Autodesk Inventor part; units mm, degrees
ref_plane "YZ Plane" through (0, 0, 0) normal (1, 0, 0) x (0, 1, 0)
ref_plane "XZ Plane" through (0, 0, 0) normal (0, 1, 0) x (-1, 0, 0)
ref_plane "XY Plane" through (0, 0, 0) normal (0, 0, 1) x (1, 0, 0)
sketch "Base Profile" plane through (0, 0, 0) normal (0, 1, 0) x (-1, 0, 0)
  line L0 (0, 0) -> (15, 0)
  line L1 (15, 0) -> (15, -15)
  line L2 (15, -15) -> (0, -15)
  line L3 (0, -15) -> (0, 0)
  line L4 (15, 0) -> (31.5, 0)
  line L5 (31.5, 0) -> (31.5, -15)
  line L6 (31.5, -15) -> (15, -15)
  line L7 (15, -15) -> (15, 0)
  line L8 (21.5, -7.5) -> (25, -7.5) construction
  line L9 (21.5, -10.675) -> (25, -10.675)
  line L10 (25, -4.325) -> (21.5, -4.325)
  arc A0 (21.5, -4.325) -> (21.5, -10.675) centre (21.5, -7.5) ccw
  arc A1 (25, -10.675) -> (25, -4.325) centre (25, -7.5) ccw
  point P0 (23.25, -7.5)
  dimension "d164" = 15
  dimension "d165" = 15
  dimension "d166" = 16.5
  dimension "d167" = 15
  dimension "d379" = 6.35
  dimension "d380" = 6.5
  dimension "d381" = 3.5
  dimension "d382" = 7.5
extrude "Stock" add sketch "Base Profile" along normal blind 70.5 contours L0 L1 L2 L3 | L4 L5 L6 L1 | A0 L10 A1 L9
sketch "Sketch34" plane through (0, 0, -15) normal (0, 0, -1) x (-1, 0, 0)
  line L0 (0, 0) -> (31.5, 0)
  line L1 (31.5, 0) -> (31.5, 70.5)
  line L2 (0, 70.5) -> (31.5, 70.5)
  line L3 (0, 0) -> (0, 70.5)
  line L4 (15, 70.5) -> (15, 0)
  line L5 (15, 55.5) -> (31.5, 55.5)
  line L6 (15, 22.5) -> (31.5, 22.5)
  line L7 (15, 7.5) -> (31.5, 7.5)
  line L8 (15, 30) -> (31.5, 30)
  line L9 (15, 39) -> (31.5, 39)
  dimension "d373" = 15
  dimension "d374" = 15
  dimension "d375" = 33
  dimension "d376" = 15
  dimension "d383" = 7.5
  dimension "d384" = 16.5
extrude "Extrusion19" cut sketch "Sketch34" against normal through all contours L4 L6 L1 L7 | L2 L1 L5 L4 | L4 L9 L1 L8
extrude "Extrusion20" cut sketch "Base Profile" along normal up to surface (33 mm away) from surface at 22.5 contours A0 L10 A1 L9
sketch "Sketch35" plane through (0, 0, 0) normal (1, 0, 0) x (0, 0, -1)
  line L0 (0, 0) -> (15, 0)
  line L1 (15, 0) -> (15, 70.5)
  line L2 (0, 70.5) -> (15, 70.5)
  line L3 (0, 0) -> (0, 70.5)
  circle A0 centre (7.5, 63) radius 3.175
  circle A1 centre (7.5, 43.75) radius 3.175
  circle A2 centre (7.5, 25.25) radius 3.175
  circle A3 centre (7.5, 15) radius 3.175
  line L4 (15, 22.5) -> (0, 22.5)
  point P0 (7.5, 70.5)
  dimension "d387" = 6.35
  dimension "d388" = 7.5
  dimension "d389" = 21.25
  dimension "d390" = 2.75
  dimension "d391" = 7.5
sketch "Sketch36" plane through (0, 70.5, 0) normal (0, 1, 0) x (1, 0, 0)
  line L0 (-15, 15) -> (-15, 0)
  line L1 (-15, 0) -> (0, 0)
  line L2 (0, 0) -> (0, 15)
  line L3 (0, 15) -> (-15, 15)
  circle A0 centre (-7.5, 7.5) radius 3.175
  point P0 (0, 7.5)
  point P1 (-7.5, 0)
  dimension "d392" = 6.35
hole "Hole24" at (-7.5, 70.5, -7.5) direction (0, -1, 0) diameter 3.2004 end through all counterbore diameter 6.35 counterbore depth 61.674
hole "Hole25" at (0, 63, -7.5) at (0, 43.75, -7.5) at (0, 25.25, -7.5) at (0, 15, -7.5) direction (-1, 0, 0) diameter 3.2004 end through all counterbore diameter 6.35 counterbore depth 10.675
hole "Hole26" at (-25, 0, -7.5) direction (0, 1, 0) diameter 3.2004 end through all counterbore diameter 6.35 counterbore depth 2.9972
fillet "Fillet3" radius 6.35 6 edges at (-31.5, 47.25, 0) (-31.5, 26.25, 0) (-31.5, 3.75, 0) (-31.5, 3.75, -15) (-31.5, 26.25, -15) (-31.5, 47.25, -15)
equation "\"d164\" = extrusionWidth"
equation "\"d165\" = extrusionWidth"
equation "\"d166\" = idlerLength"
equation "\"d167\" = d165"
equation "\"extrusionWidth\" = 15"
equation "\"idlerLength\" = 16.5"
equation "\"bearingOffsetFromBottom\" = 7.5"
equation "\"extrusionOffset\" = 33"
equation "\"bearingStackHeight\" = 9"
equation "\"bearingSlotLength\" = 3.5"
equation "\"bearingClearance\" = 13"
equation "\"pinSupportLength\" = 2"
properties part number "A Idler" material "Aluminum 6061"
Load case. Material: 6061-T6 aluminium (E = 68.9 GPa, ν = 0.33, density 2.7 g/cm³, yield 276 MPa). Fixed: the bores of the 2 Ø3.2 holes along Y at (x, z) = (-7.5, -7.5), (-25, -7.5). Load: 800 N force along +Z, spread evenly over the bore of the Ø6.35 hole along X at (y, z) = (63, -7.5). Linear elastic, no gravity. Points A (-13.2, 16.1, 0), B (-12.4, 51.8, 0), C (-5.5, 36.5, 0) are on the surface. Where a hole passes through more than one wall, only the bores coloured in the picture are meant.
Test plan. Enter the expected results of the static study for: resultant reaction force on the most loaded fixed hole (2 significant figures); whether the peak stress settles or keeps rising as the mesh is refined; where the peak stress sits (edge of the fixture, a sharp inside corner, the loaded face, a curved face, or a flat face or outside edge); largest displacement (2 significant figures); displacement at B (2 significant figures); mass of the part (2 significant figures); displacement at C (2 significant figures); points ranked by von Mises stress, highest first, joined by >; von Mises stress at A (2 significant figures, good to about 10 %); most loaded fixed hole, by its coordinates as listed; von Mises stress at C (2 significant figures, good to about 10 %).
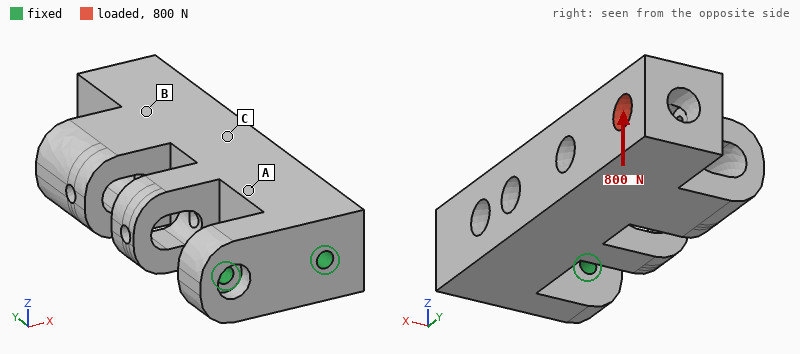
980 N
keeps rising
edge of the fixture
0.41 mm
0.26 mm
51 g
0.16 mm
A > C > B
72 MPa
(-7.5, -7.5)
42 MPa
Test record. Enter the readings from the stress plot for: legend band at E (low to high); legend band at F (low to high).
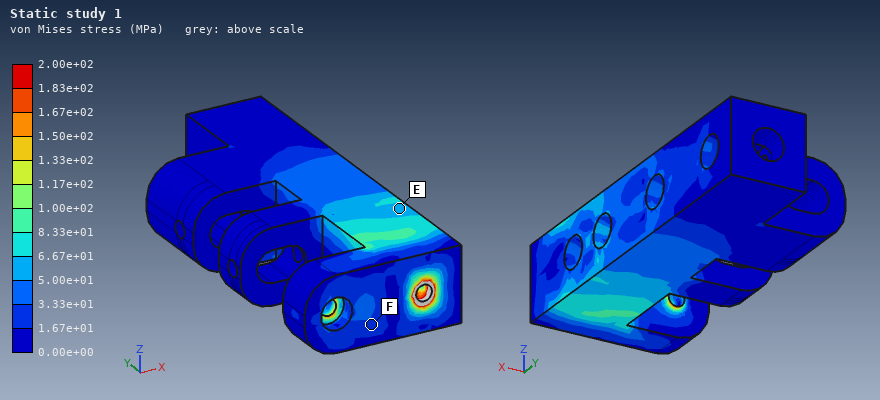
5.00e+01 to 6.67e+01 MPa
1.67e+01 to 3.33e+01 MPa
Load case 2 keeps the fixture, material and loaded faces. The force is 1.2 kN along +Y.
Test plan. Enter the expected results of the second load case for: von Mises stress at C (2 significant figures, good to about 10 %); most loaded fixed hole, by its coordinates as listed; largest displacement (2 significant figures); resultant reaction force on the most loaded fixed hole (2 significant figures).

13 MPa
(-7.5, -7.5)
73 µm
1.3 kN
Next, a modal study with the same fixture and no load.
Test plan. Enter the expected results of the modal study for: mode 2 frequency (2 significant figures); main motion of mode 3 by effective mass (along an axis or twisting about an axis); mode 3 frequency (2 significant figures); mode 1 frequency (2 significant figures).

1900 Hz
twisting about Y
5500 Hz
1900 Hz
